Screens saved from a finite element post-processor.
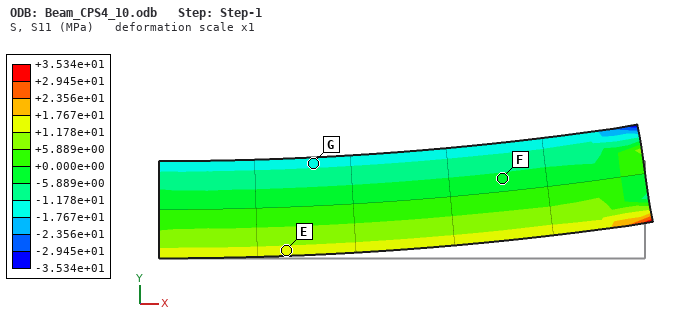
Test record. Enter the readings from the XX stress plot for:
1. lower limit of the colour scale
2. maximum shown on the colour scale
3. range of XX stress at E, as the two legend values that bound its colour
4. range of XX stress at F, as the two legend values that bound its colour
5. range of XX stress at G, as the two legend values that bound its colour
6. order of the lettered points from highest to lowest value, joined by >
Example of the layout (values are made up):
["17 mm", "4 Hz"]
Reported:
["-3.534e+01 MPa", "+3.534e+01 MPa", "+1.178e+01 to +1.767e+01 MPa", "-5.889e+00 to +0.000e+00 MPa", "-1.767e+01 to -1.178e+01 MPa", "E > F > G"]
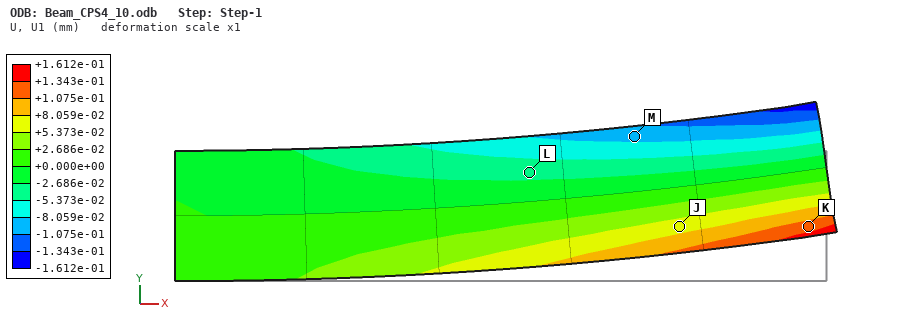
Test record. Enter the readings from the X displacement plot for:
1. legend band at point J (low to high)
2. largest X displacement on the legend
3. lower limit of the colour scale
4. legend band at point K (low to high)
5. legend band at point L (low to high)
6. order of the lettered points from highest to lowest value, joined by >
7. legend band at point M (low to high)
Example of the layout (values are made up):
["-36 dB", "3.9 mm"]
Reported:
["+5.373e-02 to +8.059e-02 mm", "+1.612e-01 mm", "-1.612e-01 mm", "+1.075e-01 to +1.343e-01 mm", "-5.373e-02 to -2.686e-02 mm", "K > J > L > M", "-1.075e-01 to -8.059e-02 mm"]
